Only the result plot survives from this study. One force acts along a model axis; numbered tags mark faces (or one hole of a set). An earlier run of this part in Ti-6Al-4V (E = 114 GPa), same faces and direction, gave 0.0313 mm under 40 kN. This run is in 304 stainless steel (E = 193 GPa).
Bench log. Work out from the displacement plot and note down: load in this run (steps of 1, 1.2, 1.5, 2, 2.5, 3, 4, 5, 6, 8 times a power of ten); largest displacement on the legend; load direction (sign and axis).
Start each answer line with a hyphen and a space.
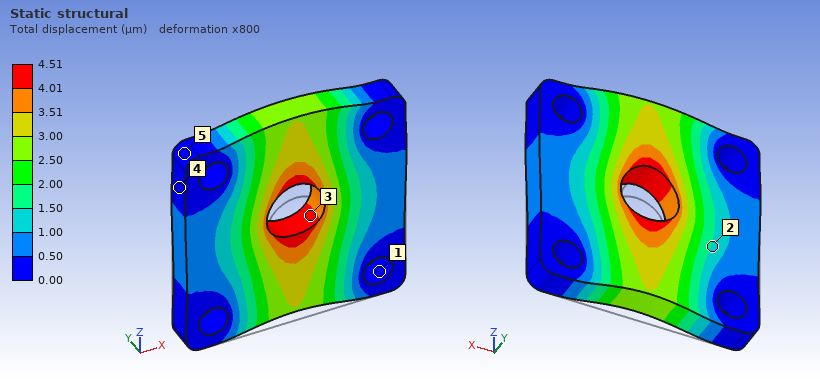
- 10 kN
- 4.51 µm
- +Z
